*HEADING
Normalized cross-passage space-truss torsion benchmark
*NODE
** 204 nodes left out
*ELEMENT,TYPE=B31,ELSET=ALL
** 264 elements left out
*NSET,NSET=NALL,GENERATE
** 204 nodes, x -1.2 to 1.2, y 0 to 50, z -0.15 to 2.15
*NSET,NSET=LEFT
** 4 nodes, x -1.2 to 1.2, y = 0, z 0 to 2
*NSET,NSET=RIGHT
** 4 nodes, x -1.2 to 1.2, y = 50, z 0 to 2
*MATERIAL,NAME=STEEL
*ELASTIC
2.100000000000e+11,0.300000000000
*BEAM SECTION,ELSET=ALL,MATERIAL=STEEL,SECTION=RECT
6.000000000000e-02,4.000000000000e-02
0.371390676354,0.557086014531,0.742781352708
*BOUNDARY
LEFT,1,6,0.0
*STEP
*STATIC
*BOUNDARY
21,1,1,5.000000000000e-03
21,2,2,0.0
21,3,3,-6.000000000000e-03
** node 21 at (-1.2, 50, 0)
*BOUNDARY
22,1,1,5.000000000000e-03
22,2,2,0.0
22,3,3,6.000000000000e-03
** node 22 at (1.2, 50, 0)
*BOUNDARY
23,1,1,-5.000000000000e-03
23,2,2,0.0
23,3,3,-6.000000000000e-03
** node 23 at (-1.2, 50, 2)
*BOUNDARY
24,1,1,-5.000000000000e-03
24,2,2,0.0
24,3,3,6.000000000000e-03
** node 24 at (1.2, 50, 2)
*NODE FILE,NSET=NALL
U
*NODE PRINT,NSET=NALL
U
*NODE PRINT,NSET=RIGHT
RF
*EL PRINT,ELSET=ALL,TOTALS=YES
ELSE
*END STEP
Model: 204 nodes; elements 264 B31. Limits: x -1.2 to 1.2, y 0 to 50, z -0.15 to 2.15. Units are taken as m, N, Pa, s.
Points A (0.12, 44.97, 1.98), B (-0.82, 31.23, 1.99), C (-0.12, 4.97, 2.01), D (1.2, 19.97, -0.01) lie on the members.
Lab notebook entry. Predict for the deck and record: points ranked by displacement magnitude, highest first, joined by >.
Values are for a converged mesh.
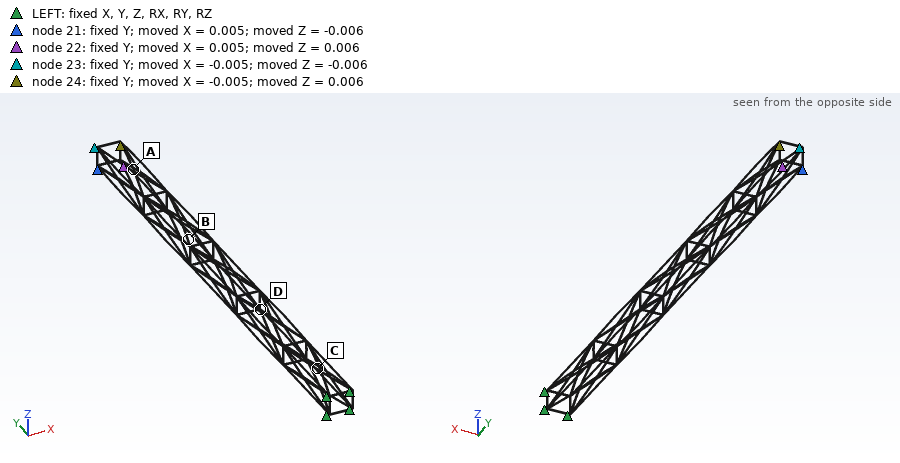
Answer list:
C > B > D > A
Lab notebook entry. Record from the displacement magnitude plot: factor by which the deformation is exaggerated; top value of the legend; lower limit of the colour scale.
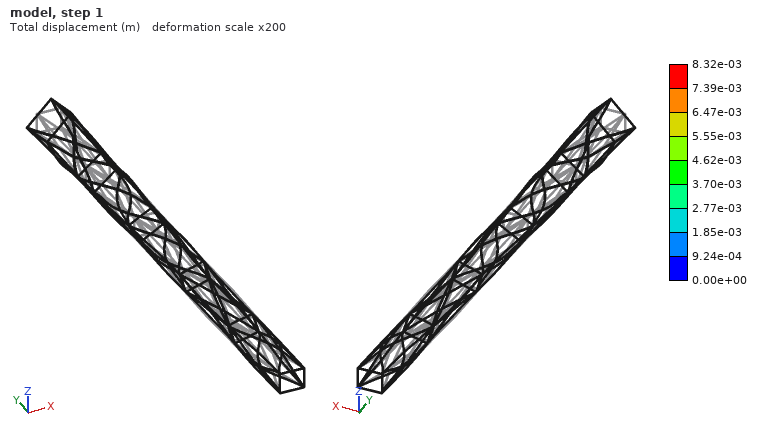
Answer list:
200
8.32e-03 m
0.00e+00 m
